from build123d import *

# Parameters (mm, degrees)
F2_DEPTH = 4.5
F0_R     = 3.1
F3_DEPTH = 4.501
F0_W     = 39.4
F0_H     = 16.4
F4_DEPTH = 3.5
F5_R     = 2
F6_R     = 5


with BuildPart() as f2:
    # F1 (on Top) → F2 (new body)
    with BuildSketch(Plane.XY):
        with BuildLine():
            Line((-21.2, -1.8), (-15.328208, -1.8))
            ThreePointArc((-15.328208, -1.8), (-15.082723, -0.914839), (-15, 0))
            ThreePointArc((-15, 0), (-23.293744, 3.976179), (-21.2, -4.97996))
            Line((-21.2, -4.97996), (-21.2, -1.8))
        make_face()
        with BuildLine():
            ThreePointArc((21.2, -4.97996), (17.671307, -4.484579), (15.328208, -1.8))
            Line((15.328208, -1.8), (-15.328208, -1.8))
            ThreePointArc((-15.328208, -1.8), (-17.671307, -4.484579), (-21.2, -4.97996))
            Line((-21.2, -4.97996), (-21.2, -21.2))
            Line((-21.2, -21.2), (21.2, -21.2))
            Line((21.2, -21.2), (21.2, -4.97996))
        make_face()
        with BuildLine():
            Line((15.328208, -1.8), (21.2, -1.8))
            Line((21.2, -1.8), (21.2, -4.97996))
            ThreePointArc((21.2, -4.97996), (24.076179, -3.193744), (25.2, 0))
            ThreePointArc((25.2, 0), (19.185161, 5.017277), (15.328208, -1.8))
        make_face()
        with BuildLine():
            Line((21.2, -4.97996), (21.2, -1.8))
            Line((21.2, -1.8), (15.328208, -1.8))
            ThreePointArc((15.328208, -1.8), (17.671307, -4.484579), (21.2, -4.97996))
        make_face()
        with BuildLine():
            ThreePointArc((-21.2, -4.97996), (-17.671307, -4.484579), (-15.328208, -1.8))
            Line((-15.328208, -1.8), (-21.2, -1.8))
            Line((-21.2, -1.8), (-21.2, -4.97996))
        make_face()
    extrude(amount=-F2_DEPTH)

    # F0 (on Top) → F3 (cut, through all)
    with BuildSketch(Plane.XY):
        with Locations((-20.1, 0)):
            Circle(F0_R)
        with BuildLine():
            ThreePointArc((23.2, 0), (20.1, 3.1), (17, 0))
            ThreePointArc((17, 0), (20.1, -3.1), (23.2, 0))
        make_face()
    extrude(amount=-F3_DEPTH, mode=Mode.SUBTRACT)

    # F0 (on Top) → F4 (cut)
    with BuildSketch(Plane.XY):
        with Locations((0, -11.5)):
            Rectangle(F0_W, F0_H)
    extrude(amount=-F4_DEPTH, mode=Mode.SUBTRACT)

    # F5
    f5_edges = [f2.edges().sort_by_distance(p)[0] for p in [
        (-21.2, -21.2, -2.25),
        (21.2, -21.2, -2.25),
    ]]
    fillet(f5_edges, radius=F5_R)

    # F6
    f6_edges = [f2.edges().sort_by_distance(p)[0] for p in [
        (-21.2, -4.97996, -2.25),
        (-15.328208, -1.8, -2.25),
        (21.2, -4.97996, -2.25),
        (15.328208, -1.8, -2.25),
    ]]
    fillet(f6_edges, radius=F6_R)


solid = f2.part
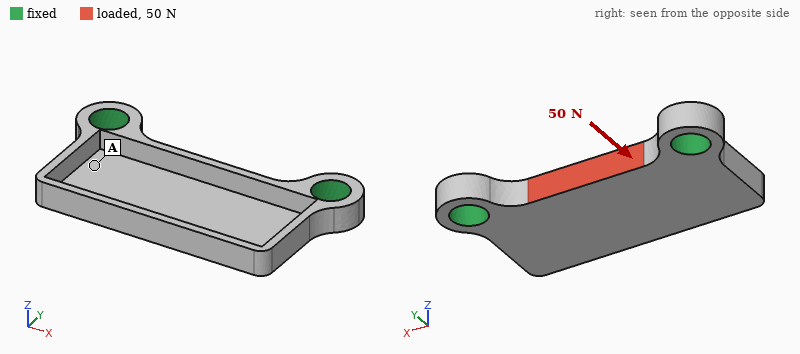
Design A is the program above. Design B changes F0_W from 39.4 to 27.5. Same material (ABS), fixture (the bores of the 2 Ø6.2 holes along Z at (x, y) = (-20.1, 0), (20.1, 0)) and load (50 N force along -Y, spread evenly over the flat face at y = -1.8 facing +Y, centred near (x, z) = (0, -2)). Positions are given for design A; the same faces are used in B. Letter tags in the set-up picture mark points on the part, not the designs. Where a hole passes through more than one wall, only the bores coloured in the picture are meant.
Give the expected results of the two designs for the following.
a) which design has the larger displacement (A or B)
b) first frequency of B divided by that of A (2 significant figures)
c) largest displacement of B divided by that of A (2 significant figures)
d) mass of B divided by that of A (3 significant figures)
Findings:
A
1.6
0.90
1.38
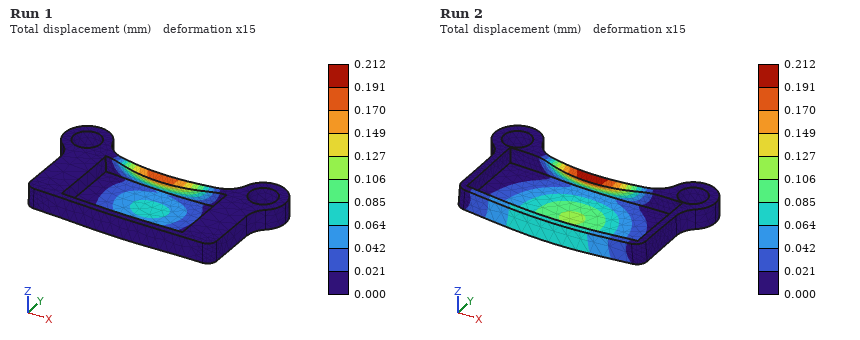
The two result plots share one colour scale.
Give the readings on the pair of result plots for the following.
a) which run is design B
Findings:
Run 1
